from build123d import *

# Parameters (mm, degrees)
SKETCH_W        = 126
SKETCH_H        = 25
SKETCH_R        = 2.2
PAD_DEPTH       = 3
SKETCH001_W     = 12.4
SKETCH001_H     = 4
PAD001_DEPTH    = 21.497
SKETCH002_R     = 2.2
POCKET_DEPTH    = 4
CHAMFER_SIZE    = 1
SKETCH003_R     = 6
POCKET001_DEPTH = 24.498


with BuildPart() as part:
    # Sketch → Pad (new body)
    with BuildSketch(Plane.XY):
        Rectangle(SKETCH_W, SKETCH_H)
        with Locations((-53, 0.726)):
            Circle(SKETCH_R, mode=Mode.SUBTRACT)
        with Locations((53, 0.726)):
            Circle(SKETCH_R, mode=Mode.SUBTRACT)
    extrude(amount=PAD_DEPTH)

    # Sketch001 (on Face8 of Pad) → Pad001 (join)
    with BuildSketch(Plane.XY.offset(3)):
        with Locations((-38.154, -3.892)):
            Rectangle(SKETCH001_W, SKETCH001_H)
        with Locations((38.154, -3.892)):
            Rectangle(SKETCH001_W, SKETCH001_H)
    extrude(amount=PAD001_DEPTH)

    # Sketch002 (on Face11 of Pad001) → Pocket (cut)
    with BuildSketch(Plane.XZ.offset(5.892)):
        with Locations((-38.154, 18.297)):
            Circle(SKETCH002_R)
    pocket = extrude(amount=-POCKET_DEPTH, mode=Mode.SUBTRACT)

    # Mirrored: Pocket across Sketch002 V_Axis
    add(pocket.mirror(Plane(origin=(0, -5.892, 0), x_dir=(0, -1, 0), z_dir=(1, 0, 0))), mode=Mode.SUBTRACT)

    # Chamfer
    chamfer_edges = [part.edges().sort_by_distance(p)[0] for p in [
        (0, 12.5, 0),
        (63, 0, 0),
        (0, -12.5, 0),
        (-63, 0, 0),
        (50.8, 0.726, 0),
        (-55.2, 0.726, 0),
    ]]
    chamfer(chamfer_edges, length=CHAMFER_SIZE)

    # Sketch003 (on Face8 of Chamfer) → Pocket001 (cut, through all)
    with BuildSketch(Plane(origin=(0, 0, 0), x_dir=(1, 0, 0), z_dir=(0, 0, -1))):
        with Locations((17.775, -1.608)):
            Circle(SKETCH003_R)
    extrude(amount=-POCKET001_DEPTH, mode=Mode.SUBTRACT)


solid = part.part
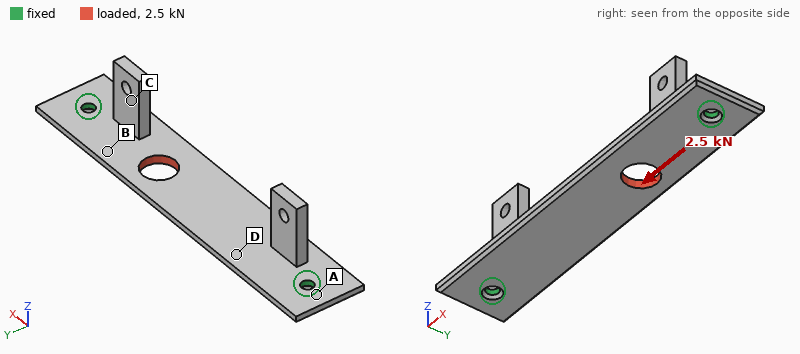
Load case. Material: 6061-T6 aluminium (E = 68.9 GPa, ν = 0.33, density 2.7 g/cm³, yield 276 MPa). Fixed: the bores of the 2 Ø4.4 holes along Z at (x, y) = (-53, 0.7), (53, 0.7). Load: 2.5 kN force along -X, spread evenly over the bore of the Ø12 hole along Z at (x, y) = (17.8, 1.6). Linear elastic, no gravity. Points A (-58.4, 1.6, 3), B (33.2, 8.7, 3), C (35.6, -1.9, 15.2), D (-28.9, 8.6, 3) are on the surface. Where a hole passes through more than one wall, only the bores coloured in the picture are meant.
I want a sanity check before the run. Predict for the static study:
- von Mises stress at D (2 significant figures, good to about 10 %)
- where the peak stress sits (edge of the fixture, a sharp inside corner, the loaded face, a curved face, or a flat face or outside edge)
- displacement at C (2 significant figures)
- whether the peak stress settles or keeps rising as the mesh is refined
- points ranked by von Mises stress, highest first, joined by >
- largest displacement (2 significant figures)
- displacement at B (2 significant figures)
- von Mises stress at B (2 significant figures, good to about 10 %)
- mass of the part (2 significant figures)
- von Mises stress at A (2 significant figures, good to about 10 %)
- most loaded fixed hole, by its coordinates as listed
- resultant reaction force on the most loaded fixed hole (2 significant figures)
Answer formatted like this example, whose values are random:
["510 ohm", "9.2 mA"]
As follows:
["15 MPa", "edge of the fixture", "5.1 µm", "keeps rising", "B > D > A > C", "17 µm", "9.9 µm", "24 MPa", "29 g", "8.4 MPa", "(53, 0.7)", "1.6 kN"]
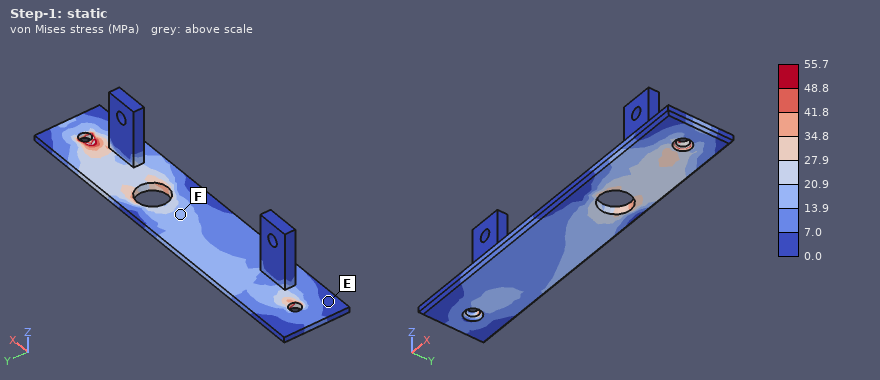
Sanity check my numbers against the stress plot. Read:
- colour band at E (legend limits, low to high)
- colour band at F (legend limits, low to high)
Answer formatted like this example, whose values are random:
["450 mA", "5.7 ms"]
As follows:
["0.0 to 7.0 MPa", "13.9 to 20.9 MPa"]
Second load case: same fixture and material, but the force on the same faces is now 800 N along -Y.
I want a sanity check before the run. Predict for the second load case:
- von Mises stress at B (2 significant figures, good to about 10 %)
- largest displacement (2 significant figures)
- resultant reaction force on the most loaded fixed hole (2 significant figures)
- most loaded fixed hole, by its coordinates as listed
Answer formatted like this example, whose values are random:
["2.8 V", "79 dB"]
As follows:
["17 MPa", "55 µm", "560 N", "(53, 0.7)"]
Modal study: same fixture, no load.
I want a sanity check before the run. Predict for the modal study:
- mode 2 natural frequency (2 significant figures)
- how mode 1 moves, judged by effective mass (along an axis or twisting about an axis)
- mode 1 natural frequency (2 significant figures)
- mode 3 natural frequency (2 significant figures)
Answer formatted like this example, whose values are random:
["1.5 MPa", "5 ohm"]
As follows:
["2800 Hz", "along Z", "1300 Hz", "3000 Hz"]
